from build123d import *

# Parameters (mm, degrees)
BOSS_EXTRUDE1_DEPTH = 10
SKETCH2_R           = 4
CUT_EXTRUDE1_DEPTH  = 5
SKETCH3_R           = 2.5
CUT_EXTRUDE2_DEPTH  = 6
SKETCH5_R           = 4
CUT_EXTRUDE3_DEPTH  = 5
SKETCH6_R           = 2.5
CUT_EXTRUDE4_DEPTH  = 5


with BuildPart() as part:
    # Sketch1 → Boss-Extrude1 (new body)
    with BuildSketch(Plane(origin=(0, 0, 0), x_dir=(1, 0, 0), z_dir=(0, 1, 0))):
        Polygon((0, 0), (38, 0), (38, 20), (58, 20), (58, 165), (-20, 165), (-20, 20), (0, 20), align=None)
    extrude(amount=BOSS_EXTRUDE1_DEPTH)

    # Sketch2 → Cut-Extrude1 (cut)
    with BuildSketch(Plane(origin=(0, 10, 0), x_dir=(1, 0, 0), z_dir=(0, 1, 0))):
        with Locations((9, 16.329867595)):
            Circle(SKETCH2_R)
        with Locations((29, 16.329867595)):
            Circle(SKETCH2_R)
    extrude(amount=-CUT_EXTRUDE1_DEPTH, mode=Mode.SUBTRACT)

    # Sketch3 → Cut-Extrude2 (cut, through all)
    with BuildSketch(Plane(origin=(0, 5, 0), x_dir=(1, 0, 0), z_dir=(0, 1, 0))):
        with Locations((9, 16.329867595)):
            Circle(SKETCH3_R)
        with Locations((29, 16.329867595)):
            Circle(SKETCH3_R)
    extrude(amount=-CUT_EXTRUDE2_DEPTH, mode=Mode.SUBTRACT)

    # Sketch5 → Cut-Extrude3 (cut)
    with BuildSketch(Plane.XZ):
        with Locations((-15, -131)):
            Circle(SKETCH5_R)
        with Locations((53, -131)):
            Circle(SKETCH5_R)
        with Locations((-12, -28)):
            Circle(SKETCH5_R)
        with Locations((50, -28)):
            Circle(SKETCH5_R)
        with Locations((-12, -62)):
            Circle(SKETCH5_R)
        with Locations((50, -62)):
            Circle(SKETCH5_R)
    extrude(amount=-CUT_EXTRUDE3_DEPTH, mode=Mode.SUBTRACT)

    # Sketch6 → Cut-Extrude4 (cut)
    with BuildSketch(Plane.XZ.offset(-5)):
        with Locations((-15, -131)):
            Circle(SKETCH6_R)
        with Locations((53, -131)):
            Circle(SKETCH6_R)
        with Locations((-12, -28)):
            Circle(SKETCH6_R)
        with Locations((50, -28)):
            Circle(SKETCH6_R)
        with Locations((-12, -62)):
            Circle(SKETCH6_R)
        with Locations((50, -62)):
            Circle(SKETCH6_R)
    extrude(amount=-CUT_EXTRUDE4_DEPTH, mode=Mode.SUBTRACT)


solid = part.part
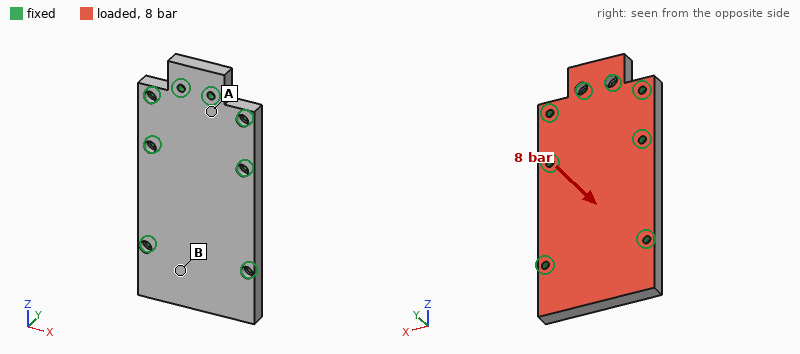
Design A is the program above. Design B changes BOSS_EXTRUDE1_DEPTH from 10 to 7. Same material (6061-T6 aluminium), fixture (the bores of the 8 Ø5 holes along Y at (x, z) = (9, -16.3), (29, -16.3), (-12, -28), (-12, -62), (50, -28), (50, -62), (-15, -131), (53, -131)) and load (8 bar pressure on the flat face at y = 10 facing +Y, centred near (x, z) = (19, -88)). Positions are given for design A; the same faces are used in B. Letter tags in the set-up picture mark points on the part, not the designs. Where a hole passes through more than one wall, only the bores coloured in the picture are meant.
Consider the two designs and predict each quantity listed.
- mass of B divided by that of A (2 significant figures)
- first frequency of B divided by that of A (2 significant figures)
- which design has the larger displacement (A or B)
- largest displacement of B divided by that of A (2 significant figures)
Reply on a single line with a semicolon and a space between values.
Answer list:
0.70; 0.70; B; 2.9
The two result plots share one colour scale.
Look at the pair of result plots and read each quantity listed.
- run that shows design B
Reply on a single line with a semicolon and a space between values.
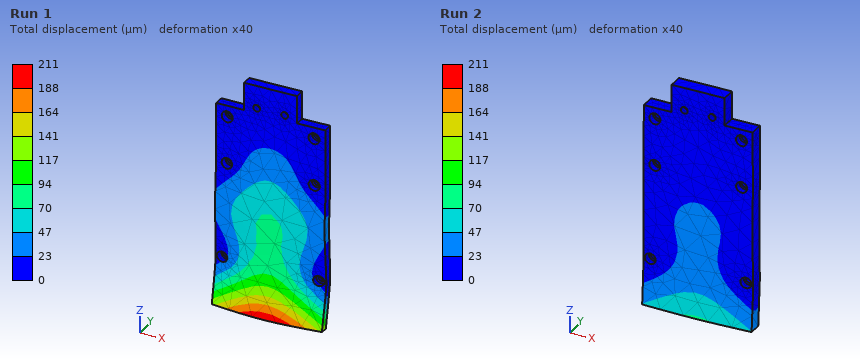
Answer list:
Run 1
